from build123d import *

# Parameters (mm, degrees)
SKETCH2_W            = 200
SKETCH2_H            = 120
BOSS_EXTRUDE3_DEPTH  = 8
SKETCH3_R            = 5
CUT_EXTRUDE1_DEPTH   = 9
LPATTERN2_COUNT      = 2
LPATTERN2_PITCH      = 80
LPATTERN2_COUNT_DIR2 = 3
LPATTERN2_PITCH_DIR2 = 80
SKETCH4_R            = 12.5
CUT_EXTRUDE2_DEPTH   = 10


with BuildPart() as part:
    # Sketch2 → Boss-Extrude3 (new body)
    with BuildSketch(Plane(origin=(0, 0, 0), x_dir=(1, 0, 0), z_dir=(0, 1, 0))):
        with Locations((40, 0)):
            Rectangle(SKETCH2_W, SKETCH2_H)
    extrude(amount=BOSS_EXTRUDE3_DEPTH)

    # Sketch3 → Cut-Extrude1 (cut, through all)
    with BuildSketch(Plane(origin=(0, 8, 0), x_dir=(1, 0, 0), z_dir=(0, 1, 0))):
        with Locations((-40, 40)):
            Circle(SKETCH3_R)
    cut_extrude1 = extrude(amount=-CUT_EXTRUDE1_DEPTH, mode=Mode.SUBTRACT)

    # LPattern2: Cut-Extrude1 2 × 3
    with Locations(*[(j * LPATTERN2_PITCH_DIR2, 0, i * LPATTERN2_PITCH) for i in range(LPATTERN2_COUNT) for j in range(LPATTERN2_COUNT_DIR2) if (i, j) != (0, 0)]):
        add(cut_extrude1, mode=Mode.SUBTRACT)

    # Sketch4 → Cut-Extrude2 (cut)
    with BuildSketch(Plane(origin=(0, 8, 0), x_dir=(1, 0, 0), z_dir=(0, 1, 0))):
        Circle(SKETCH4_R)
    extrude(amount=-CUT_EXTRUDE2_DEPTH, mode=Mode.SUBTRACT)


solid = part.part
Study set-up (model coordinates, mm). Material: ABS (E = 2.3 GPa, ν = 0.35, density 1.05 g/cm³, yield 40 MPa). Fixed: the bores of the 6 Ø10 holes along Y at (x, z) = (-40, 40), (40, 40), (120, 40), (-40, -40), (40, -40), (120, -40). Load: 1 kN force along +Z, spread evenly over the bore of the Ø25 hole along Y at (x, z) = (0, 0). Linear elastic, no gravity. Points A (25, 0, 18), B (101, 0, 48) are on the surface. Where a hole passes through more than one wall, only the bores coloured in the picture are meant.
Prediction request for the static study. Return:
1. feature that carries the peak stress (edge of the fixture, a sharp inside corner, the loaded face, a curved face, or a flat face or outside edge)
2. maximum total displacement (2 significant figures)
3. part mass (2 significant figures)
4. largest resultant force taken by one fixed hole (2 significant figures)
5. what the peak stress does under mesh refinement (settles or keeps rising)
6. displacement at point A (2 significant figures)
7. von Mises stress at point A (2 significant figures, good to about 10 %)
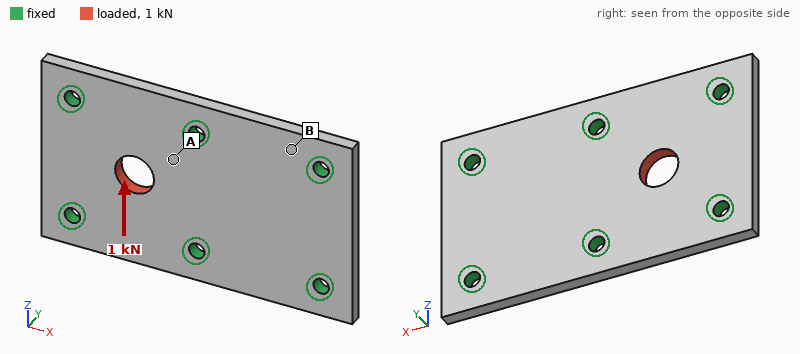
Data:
edge of the fixture
32 µm
190 g
270 N
keeps rising
14 µm
1.1 MPa
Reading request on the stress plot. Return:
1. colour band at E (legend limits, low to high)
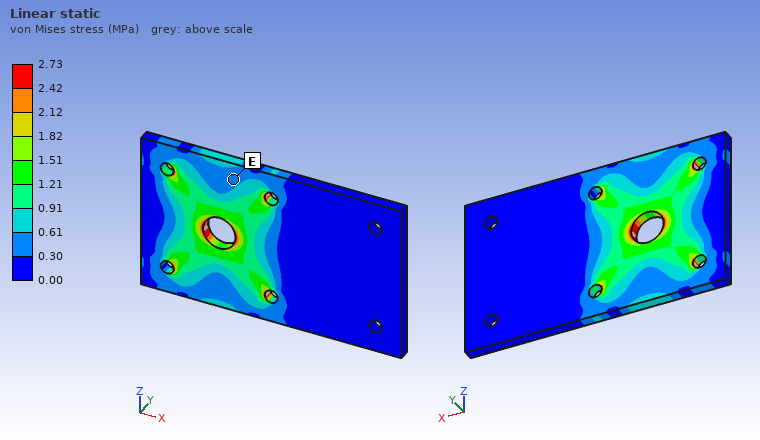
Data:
0.30 to 0.61 MPa
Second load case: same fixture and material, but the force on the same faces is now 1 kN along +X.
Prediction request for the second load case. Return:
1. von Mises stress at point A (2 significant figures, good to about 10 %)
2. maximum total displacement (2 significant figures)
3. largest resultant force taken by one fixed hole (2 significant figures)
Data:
1.1 MPa
32 µm
250 N
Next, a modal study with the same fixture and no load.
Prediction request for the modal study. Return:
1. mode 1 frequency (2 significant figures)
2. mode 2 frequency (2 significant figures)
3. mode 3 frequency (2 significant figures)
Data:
1400 Hz
1500 Hz
1900 Hz
